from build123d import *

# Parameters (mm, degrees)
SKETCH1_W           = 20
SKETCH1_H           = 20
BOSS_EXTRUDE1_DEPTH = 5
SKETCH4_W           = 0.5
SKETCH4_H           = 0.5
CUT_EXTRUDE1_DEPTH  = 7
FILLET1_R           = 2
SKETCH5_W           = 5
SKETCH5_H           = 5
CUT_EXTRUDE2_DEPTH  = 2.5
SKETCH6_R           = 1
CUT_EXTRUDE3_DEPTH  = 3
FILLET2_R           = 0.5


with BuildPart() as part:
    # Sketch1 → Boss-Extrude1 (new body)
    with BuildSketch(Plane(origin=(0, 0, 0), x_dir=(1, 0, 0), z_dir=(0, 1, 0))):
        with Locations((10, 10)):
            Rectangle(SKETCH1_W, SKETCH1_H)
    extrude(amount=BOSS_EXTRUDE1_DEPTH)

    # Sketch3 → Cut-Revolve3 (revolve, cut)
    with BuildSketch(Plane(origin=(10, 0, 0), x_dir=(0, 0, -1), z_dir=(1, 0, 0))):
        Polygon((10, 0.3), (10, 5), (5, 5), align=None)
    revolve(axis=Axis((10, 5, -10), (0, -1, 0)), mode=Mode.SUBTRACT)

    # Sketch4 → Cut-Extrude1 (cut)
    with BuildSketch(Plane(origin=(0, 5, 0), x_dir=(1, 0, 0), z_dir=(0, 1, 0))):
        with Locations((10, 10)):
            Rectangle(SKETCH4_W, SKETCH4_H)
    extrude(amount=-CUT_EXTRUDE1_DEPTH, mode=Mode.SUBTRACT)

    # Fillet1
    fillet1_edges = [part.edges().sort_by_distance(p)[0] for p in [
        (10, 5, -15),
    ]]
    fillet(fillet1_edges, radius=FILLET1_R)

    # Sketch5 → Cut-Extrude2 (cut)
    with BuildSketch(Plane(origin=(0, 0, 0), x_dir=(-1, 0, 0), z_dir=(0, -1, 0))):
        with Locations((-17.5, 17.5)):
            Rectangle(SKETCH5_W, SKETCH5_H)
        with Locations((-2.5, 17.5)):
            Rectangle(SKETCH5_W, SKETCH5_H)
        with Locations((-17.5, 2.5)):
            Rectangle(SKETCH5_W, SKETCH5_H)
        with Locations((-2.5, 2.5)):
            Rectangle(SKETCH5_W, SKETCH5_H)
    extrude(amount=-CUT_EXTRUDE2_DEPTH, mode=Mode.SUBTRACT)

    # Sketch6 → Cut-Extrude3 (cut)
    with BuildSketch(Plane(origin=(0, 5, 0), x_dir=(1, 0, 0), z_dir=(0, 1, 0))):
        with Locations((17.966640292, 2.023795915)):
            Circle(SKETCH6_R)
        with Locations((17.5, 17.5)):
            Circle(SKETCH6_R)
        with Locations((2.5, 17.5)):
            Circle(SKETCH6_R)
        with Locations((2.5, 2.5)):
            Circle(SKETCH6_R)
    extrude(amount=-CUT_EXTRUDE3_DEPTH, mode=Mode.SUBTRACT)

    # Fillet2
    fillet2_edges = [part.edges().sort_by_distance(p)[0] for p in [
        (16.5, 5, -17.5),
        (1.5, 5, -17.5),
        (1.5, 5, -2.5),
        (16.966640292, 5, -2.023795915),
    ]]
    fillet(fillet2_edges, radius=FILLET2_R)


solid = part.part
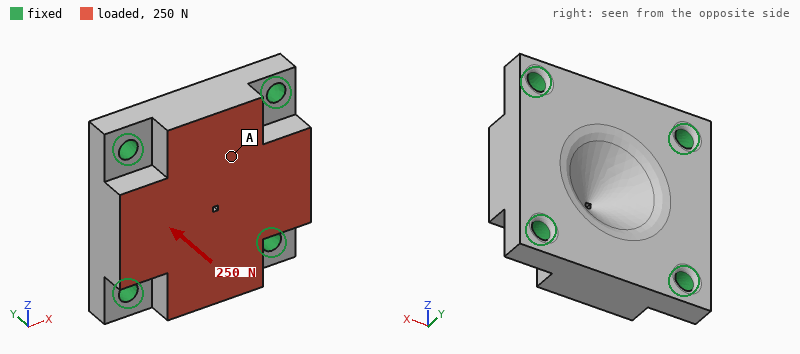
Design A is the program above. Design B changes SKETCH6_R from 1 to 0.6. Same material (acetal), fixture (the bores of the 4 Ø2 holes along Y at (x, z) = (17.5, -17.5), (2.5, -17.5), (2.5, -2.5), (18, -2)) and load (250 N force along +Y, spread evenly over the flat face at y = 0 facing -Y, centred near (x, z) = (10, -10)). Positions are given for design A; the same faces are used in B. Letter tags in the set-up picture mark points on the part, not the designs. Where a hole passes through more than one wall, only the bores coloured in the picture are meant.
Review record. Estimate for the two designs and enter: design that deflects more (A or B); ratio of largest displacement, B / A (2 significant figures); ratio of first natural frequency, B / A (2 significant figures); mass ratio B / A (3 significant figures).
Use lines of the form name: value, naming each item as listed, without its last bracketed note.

design that deflects more: B
ratio of largest displacement, B / A: 1.3
ratio of first natural frequency, B / A: 0.87
mass ratio B / A: 1.01
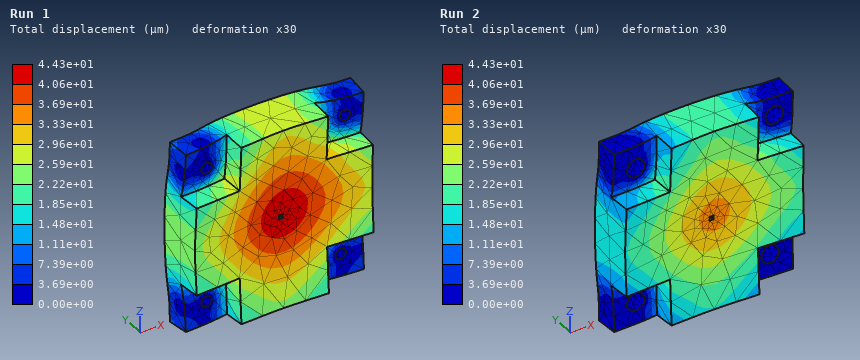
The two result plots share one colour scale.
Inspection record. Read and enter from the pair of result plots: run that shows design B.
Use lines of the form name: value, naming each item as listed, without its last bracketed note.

run that shows design B: Run 1
